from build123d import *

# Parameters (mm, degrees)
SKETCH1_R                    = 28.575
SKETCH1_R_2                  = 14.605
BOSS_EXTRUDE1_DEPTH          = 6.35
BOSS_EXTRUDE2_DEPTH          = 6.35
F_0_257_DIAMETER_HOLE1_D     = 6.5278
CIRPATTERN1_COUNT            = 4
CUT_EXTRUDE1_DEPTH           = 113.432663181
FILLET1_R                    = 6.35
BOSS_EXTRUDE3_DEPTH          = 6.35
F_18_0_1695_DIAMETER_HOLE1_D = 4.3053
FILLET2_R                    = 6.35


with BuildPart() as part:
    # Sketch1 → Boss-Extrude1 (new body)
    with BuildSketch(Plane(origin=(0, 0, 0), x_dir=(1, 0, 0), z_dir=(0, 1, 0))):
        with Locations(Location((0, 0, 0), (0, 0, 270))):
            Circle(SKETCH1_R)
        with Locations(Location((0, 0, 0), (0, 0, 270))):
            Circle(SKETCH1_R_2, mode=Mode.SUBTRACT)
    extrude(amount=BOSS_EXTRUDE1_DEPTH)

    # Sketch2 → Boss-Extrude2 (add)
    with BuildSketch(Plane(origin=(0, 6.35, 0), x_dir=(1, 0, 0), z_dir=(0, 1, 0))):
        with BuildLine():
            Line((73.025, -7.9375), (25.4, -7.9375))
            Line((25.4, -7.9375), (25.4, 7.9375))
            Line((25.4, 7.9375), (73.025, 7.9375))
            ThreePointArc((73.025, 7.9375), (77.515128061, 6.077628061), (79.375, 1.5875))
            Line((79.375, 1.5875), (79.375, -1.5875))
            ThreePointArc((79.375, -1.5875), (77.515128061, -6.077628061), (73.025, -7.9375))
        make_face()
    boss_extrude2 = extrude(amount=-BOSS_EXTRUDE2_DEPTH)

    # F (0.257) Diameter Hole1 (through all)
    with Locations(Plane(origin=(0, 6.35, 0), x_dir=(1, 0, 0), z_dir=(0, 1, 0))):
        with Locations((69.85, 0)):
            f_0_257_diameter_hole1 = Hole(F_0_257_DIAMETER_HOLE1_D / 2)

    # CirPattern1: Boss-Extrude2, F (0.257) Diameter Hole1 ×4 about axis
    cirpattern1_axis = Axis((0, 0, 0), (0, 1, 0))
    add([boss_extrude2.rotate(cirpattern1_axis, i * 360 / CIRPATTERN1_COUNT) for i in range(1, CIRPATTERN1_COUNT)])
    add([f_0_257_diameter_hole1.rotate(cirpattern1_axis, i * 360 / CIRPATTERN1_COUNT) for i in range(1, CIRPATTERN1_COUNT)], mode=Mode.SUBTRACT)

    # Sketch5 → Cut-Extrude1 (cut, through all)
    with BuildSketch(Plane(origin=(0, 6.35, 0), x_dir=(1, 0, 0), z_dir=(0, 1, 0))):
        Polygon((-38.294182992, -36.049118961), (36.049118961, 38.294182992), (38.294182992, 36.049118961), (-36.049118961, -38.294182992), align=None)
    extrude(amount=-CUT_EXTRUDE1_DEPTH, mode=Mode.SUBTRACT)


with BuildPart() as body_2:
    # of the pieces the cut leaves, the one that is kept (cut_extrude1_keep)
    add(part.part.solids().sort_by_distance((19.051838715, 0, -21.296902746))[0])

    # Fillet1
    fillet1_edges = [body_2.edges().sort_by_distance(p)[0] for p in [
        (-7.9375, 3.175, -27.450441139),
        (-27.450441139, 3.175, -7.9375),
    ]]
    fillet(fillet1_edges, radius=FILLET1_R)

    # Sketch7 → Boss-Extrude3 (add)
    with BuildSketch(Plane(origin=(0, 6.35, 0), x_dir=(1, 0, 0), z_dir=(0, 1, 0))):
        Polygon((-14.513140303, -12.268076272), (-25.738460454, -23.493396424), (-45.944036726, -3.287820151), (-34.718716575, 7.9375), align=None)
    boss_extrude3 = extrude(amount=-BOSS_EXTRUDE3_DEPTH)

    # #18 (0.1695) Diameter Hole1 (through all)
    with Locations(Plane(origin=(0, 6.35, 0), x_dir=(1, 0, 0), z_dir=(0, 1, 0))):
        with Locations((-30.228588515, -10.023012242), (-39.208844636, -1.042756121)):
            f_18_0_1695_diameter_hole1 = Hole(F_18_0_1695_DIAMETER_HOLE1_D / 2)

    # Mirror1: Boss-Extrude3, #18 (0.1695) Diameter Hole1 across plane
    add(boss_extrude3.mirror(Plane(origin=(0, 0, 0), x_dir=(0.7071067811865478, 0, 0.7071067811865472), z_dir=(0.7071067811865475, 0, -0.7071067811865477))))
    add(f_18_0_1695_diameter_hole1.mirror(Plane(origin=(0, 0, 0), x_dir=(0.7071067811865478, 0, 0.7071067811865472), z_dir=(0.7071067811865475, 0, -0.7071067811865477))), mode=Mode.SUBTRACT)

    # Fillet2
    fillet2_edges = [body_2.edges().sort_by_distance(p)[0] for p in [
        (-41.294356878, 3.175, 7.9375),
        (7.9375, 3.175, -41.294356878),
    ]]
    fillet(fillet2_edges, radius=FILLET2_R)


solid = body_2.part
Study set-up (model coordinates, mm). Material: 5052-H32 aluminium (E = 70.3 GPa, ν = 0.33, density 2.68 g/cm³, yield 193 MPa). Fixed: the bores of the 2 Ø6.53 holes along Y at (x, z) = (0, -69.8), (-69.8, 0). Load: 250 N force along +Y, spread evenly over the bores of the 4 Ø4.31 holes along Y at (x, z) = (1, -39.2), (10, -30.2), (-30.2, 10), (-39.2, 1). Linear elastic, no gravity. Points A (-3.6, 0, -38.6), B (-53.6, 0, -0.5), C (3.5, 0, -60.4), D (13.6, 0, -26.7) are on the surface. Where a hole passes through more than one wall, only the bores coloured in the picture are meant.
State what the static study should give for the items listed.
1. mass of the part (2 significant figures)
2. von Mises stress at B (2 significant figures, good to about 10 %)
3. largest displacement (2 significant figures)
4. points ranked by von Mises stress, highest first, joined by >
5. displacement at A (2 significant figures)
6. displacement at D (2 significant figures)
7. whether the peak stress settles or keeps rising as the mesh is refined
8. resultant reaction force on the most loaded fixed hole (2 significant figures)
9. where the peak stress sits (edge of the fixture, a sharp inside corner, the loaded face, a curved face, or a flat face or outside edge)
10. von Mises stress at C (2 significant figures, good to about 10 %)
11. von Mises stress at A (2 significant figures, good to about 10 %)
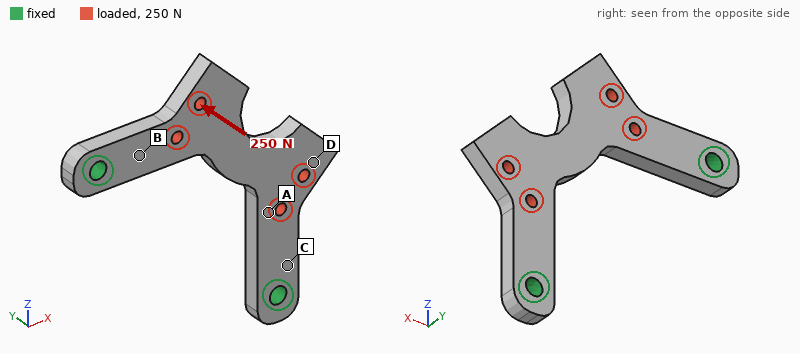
45 g
21 MPa
0.12 mm
C > B > A > D
0.043 mm
0.094 mm
keeps rising
130 N
edge of the fixture
28 MPa
10 MPa
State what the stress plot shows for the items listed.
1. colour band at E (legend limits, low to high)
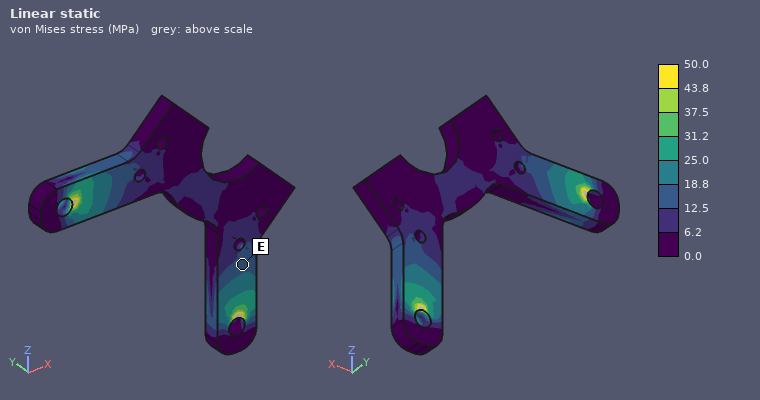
12.5 to 18.8 MPa
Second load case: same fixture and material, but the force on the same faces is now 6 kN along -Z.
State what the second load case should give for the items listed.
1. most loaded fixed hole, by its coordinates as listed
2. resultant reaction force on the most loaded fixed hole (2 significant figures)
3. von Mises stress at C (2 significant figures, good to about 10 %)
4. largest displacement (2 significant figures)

(0, -69.8)
4.6 kN
54 MPa
60 µm
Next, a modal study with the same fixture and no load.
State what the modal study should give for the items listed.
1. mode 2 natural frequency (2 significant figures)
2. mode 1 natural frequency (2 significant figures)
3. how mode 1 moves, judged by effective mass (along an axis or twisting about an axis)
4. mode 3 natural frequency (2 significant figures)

3300 Hz
1500 Hz
along Y
5700 Hz
